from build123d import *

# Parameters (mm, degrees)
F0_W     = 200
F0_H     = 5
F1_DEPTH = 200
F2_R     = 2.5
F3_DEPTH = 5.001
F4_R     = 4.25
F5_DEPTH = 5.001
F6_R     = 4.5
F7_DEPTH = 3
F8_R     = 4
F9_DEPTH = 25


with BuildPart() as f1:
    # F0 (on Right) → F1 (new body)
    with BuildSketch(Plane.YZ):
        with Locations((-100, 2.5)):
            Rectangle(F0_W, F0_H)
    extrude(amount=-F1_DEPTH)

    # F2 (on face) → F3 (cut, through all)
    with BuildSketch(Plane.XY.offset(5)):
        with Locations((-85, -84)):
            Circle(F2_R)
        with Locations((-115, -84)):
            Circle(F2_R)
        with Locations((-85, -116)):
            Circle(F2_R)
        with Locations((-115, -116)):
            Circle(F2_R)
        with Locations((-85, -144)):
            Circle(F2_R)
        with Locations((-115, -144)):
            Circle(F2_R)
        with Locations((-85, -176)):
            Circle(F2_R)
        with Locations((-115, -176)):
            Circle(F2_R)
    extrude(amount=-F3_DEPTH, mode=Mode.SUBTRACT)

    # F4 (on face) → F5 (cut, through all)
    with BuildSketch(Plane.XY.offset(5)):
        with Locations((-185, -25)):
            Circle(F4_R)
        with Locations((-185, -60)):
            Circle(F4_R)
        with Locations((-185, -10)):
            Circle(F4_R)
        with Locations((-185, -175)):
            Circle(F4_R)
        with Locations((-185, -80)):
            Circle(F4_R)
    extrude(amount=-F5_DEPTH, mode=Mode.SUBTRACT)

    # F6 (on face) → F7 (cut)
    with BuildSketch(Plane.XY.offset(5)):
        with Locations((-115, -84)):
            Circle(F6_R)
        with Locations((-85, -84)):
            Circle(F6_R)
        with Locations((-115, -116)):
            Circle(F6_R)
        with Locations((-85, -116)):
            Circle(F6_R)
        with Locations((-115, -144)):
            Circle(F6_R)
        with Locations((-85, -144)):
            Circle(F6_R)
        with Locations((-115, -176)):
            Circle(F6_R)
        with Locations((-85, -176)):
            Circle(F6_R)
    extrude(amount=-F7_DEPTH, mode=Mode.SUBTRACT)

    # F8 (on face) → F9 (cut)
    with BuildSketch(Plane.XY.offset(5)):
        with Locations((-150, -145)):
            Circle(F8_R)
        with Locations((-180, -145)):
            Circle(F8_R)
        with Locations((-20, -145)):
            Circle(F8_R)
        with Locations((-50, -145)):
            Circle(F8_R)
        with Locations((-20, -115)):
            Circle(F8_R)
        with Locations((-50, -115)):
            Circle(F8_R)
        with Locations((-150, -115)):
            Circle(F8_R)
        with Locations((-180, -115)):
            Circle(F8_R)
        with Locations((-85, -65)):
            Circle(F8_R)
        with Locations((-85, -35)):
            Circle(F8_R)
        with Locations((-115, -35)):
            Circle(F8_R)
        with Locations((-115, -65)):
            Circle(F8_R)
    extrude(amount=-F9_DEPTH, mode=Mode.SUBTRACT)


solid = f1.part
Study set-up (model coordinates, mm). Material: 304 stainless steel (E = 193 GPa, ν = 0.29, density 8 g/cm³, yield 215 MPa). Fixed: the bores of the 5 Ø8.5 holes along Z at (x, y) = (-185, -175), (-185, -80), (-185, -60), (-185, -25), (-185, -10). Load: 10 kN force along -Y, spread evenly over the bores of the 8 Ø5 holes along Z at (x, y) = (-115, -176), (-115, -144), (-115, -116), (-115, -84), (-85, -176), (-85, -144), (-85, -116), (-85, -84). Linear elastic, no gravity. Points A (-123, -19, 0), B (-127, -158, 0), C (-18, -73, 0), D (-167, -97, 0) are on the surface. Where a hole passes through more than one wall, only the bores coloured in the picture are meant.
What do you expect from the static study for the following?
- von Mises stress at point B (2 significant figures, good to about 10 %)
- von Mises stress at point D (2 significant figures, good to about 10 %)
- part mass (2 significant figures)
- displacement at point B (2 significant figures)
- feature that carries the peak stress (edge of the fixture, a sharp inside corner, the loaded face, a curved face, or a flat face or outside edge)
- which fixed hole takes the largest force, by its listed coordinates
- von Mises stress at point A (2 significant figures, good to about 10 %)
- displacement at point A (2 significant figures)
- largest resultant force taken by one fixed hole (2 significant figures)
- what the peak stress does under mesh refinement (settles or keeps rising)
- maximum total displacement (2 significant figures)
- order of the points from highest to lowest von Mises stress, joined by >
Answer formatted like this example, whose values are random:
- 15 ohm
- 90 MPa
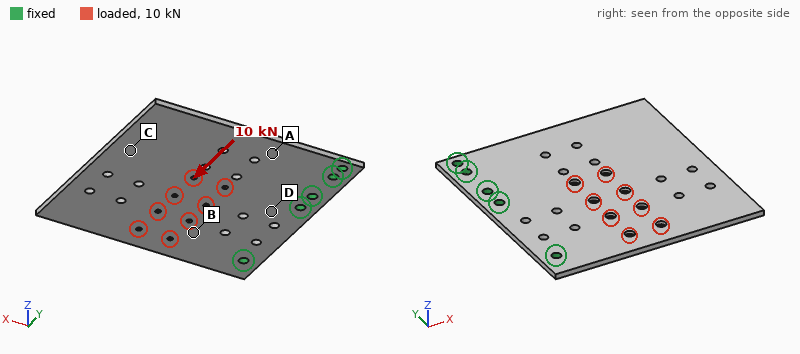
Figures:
- 32 MPa
- 23 MPa
- 1.5 kg
- 0.032 mm
- edge of the fixture
- (-185, -175)
- 14 MPa
- 0.030 mm
- 6.2 kN
- keeps rising
- 0.13 mm
- B > D > A > C
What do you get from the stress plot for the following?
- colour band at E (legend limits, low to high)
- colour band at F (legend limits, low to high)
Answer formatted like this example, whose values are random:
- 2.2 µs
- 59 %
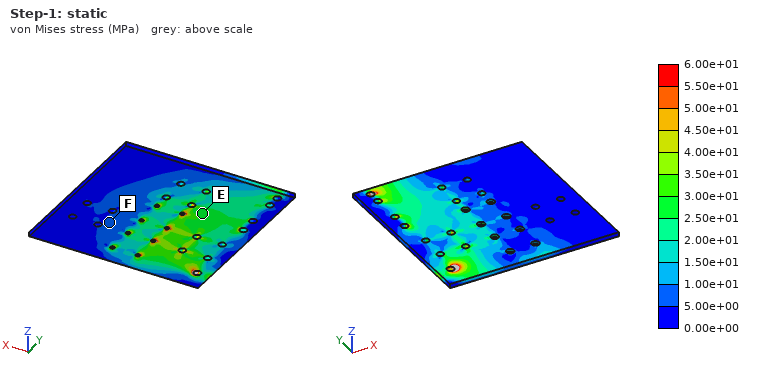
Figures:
- 2.50e+01 to 3.00e+01 MPa
- 5.00e+00 to 1.00e+01 MPa
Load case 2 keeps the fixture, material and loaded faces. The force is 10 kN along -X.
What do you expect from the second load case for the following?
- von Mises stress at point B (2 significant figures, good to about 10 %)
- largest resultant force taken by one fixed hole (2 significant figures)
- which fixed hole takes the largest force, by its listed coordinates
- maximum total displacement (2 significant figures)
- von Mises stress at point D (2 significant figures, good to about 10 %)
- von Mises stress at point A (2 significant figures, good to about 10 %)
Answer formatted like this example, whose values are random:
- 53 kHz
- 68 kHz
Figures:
- 34 MPa
- 5.8 kN
- (-185, -175)
- 0.52 mm
- 28 MPa
- 15 MPa
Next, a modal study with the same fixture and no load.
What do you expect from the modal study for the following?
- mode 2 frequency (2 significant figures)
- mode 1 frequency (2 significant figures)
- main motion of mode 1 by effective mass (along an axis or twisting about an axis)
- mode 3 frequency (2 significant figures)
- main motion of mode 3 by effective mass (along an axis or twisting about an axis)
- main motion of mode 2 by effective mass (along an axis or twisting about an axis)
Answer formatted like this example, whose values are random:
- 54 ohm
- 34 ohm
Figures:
- 270 Hz
- 110 Hz
- along Z
- 700 Hz
- along Z
- twisting about X
